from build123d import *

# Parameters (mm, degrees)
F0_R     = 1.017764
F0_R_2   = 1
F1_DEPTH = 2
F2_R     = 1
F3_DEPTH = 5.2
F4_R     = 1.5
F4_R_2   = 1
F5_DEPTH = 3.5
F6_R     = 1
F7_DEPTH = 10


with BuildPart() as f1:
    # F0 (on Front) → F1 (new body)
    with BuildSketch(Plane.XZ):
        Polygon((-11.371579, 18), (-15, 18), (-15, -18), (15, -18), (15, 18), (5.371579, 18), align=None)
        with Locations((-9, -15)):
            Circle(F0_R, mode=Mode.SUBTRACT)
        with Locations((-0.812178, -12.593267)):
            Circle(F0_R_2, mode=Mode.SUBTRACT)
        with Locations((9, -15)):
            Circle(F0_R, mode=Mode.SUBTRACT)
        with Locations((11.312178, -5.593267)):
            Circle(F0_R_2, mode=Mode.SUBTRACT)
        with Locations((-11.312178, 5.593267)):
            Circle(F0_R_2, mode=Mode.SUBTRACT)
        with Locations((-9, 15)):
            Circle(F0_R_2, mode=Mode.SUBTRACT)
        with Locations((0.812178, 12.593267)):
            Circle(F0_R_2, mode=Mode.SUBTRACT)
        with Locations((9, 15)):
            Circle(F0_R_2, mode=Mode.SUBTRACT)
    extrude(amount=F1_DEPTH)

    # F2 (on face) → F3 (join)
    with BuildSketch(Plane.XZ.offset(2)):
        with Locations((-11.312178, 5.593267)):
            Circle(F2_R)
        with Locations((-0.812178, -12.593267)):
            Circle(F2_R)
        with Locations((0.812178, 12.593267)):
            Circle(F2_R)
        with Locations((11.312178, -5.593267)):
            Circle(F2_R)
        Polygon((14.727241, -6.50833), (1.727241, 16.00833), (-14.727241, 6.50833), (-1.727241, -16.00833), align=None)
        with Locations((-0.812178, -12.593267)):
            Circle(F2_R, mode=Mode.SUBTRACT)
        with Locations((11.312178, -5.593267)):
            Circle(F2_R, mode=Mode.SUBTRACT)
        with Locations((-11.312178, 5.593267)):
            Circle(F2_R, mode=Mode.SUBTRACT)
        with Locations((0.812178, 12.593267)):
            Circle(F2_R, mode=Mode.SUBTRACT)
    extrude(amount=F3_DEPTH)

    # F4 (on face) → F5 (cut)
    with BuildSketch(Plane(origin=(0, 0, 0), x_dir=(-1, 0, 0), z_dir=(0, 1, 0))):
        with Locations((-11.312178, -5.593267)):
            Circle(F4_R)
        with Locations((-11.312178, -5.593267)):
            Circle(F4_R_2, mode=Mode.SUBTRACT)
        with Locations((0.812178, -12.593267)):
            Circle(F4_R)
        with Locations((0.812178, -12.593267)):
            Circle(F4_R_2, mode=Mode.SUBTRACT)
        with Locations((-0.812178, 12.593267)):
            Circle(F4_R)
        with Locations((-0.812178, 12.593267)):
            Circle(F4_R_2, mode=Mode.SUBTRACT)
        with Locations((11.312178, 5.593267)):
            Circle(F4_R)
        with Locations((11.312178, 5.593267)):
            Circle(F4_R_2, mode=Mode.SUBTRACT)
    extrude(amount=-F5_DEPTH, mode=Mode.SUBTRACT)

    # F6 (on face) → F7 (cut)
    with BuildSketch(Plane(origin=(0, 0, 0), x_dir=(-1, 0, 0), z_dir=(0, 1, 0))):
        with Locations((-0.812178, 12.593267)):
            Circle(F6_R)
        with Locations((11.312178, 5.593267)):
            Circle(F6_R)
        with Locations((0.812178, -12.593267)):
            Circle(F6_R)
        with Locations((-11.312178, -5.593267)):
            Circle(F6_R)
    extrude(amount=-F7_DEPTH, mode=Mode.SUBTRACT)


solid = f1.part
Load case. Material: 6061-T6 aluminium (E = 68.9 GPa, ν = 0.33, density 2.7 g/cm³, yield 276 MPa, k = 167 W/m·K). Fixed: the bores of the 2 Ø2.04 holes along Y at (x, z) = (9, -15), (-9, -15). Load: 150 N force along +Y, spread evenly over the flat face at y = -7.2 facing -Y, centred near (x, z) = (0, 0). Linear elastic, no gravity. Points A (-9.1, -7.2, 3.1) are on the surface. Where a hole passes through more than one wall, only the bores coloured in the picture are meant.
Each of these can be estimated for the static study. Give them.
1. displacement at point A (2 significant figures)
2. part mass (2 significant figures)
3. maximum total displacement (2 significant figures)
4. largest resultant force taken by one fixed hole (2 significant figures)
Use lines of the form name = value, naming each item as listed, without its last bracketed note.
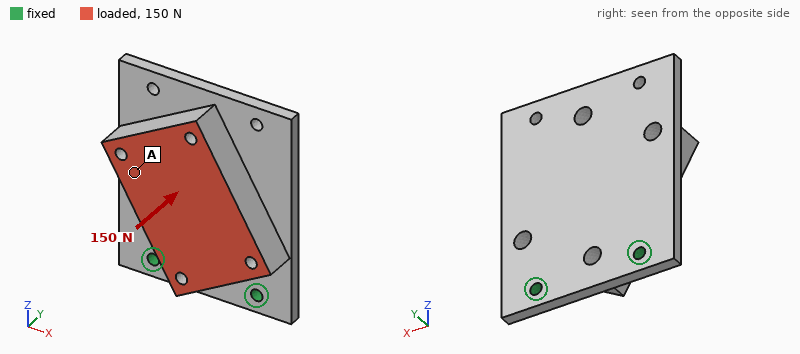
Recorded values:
displacement at point A = 0.13 mm
part mass = 12 g
maximum total displacement = 0.23 mm
largest resultant force taken by one fixed hole = 78 N
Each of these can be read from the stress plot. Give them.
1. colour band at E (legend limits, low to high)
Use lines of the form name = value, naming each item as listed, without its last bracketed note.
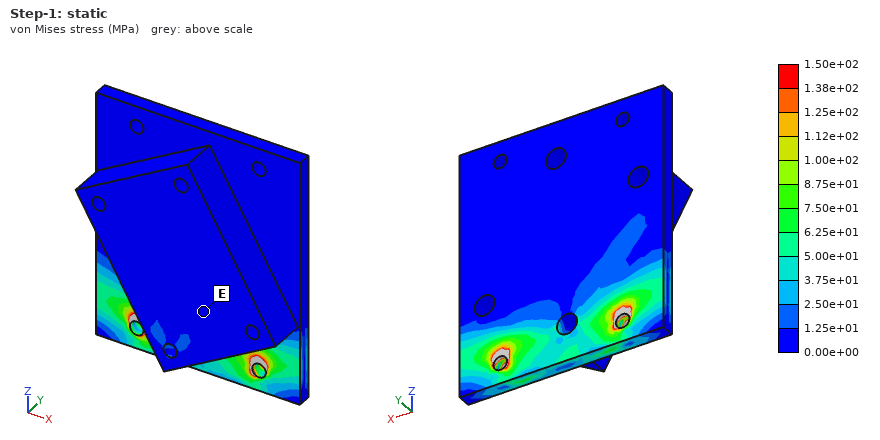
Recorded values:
colour band at E = 0.00e+00 to 1.25e+01 MPa
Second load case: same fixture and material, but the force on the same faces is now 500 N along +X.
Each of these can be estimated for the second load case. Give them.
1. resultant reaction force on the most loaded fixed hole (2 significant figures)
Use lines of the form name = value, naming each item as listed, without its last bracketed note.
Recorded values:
resultant reaction force on the most loaded fixed hole = 500 N
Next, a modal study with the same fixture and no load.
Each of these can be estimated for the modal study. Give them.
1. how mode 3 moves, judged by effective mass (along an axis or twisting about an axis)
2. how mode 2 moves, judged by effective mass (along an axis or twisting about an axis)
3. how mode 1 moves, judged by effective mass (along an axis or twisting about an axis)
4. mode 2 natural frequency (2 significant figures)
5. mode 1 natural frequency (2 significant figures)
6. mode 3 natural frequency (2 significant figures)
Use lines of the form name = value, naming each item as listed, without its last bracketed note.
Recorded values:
how mode 3 moves, judged by effective mass = along X
how mode 2 moves, judged by effective mass = twisting about Z
how mode 1 moves, judged by effective mass = along Y
mode 2 natural frequency = 7900 Hz
mode 1 natural frequency = 1500 Hz
mode 3 natural frequency = 9800 Hz
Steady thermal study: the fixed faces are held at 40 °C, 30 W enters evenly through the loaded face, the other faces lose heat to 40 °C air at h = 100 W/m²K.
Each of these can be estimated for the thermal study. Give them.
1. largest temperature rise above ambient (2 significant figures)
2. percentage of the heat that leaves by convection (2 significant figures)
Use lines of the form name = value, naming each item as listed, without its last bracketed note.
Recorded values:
largest temperature rise above ambient = 31 K
percentage of the heat that leaves by convection = 20 %
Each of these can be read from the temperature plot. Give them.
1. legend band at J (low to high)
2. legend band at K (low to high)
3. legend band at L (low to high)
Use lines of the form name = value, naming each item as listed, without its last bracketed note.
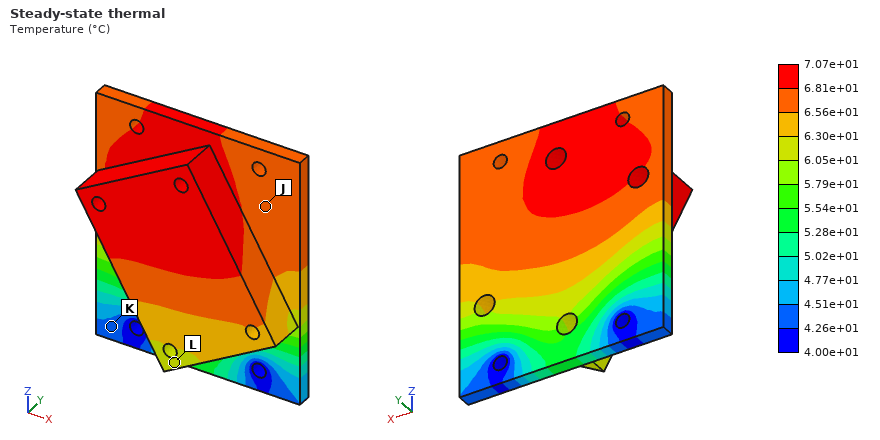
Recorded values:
legend band at J = 6.56e+01 to 6.81e+01 °C
legend band at K = 4.26e+01 to 4.51e+01 °C
legend band at L = 6.05e+01 to 6.30e+01 °C
